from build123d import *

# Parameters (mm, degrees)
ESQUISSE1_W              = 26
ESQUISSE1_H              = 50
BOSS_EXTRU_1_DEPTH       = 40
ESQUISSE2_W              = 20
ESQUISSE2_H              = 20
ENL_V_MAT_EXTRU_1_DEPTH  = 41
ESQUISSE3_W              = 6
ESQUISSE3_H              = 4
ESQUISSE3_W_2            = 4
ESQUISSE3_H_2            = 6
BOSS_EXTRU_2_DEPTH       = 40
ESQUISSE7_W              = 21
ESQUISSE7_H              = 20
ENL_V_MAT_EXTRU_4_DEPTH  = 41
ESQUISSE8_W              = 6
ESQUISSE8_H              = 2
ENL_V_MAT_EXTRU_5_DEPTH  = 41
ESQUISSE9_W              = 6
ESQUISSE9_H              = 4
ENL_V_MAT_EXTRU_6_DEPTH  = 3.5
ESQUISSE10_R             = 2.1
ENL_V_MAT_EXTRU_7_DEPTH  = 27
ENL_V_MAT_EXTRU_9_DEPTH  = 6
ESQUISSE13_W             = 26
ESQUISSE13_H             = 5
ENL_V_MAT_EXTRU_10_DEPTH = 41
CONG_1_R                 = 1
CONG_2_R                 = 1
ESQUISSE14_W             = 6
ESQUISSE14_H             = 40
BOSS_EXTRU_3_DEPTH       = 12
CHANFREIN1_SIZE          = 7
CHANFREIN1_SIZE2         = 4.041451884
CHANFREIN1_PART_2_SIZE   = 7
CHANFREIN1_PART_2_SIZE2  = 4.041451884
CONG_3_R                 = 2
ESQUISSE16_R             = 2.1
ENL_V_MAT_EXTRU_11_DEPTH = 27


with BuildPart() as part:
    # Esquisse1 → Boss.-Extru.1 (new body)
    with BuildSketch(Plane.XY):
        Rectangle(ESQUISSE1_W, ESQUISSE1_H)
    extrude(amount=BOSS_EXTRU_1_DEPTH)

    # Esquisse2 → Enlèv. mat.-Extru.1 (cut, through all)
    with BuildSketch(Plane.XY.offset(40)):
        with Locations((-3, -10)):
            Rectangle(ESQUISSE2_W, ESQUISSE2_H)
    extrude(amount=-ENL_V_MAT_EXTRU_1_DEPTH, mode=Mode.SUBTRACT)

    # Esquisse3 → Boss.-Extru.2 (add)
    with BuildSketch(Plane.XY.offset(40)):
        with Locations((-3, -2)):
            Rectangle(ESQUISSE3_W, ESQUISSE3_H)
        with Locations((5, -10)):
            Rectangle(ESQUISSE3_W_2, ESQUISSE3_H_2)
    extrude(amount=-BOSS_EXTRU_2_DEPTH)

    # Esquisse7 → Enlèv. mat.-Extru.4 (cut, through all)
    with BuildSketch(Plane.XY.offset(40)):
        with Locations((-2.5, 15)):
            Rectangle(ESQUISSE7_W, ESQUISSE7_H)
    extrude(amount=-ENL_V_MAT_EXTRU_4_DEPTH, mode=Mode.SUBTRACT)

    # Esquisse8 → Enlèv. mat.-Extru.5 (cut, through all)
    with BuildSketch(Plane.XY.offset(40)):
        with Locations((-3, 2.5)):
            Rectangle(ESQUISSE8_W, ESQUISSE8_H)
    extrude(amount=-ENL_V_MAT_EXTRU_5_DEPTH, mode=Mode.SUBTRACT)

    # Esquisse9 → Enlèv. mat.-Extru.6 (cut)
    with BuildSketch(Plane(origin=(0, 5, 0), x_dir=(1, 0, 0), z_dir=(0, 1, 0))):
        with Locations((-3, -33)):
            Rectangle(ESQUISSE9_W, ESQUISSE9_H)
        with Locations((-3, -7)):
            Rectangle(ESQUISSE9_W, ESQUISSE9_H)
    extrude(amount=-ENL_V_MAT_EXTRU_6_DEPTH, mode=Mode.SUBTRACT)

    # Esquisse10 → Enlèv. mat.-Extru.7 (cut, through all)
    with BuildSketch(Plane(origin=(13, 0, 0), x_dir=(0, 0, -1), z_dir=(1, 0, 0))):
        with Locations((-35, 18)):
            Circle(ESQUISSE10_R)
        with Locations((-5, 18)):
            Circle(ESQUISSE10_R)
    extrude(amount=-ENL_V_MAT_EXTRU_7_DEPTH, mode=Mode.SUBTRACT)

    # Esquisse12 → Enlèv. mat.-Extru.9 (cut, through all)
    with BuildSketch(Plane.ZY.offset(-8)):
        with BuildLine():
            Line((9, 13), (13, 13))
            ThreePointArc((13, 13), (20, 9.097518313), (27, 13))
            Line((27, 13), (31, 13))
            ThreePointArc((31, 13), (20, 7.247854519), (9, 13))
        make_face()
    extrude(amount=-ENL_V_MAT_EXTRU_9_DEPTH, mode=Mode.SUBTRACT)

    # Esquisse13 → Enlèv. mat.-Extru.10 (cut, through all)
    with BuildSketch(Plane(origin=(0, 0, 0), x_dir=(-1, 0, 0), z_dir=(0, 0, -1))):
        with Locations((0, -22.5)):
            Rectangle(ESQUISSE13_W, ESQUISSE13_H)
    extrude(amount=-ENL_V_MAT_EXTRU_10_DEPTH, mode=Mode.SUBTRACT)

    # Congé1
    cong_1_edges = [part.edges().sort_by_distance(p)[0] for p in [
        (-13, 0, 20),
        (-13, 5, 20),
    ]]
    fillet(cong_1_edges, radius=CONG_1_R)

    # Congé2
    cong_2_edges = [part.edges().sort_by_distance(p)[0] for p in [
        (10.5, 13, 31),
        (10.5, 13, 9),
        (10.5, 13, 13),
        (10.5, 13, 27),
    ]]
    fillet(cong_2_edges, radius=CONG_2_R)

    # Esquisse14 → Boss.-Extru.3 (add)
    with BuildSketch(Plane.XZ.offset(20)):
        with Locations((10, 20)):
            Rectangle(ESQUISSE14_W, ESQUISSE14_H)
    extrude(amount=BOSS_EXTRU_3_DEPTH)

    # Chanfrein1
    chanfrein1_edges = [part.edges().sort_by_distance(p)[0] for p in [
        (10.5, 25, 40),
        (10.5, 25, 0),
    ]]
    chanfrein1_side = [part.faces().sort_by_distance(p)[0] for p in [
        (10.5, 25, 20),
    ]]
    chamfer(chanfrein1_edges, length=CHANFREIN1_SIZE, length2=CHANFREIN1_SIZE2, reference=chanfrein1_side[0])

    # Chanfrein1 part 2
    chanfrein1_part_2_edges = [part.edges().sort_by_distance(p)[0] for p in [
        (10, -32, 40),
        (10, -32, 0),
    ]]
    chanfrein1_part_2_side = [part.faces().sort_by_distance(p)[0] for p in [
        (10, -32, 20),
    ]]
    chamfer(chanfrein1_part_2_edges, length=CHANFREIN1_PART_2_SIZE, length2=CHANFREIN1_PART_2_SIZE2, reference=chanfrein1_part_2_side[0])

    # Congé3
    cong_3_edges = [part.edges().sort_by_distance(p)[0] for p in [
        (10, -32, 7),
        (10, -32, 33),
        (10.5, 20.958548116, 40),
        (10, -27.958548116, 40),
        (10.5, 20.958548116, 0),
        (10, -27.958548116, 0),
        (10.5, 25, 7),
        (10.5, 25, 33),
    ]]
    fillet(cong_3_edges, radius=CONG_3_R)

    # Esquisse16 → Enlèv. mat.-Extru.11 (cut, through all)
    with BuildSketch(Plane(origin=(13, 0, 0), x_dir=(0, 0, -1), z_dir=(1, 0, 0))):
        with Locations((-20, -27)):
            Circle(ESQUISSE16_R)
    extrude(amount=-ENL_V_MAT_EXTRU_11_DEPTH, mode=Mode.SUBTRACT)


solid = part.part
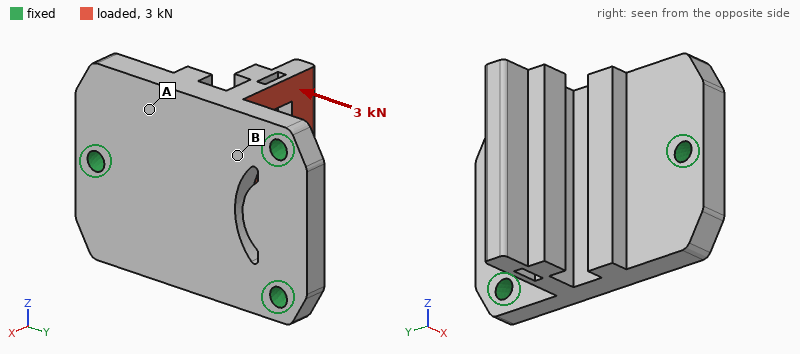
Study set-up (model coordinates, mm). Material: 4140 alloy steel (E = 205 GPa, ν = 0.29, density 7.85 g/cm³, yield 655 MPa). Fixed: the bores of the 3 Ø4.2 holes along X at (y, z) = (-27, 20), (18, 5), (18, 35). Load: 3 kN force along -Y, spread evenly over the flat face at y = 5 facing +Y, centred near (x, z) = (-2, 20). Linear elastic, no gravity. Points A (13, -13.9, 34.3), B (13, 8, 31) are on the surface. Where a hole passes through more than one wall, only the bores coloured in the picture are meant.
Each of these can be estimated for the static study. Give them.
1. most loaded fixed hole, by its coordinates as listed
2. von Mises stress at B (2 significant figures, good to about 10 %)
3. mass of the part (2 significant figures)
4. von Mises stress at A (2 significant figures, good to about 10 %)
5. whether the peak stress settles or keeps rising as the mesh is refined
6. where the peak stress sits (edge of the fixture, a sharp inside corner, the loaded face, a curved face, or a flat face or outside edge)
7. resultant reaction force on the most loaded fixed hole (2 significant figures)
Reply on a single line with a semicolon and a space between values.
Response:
(-27, 20); 55 MPa; 140 g; 18 MPa; keeps rising; edge of the fixture; 1.9 kN
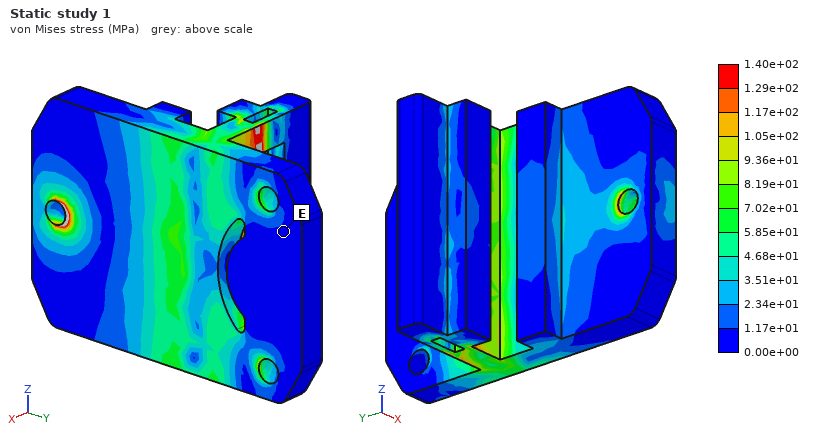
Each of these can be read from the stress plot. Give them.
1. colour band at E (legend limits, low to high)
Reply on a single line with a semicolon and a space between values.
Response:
0.00e+00 to 1.17e+01 MPa
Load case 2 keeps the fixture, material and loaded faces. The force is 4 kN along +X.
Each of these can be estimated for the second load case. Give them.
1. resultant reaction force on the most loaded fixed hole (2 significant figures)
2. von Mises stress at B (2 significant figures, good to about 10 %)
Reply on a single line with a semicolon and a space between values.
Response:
1.6 kN; 89 MPa
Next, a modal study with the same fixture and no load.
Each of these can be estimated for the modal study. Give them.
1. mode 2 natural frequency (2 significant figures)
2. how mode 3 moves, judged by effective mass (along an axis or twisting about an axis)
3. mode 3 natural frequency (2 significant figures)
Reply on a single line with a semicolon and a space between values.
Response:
6800 Hz; along X; 8600 Hz
